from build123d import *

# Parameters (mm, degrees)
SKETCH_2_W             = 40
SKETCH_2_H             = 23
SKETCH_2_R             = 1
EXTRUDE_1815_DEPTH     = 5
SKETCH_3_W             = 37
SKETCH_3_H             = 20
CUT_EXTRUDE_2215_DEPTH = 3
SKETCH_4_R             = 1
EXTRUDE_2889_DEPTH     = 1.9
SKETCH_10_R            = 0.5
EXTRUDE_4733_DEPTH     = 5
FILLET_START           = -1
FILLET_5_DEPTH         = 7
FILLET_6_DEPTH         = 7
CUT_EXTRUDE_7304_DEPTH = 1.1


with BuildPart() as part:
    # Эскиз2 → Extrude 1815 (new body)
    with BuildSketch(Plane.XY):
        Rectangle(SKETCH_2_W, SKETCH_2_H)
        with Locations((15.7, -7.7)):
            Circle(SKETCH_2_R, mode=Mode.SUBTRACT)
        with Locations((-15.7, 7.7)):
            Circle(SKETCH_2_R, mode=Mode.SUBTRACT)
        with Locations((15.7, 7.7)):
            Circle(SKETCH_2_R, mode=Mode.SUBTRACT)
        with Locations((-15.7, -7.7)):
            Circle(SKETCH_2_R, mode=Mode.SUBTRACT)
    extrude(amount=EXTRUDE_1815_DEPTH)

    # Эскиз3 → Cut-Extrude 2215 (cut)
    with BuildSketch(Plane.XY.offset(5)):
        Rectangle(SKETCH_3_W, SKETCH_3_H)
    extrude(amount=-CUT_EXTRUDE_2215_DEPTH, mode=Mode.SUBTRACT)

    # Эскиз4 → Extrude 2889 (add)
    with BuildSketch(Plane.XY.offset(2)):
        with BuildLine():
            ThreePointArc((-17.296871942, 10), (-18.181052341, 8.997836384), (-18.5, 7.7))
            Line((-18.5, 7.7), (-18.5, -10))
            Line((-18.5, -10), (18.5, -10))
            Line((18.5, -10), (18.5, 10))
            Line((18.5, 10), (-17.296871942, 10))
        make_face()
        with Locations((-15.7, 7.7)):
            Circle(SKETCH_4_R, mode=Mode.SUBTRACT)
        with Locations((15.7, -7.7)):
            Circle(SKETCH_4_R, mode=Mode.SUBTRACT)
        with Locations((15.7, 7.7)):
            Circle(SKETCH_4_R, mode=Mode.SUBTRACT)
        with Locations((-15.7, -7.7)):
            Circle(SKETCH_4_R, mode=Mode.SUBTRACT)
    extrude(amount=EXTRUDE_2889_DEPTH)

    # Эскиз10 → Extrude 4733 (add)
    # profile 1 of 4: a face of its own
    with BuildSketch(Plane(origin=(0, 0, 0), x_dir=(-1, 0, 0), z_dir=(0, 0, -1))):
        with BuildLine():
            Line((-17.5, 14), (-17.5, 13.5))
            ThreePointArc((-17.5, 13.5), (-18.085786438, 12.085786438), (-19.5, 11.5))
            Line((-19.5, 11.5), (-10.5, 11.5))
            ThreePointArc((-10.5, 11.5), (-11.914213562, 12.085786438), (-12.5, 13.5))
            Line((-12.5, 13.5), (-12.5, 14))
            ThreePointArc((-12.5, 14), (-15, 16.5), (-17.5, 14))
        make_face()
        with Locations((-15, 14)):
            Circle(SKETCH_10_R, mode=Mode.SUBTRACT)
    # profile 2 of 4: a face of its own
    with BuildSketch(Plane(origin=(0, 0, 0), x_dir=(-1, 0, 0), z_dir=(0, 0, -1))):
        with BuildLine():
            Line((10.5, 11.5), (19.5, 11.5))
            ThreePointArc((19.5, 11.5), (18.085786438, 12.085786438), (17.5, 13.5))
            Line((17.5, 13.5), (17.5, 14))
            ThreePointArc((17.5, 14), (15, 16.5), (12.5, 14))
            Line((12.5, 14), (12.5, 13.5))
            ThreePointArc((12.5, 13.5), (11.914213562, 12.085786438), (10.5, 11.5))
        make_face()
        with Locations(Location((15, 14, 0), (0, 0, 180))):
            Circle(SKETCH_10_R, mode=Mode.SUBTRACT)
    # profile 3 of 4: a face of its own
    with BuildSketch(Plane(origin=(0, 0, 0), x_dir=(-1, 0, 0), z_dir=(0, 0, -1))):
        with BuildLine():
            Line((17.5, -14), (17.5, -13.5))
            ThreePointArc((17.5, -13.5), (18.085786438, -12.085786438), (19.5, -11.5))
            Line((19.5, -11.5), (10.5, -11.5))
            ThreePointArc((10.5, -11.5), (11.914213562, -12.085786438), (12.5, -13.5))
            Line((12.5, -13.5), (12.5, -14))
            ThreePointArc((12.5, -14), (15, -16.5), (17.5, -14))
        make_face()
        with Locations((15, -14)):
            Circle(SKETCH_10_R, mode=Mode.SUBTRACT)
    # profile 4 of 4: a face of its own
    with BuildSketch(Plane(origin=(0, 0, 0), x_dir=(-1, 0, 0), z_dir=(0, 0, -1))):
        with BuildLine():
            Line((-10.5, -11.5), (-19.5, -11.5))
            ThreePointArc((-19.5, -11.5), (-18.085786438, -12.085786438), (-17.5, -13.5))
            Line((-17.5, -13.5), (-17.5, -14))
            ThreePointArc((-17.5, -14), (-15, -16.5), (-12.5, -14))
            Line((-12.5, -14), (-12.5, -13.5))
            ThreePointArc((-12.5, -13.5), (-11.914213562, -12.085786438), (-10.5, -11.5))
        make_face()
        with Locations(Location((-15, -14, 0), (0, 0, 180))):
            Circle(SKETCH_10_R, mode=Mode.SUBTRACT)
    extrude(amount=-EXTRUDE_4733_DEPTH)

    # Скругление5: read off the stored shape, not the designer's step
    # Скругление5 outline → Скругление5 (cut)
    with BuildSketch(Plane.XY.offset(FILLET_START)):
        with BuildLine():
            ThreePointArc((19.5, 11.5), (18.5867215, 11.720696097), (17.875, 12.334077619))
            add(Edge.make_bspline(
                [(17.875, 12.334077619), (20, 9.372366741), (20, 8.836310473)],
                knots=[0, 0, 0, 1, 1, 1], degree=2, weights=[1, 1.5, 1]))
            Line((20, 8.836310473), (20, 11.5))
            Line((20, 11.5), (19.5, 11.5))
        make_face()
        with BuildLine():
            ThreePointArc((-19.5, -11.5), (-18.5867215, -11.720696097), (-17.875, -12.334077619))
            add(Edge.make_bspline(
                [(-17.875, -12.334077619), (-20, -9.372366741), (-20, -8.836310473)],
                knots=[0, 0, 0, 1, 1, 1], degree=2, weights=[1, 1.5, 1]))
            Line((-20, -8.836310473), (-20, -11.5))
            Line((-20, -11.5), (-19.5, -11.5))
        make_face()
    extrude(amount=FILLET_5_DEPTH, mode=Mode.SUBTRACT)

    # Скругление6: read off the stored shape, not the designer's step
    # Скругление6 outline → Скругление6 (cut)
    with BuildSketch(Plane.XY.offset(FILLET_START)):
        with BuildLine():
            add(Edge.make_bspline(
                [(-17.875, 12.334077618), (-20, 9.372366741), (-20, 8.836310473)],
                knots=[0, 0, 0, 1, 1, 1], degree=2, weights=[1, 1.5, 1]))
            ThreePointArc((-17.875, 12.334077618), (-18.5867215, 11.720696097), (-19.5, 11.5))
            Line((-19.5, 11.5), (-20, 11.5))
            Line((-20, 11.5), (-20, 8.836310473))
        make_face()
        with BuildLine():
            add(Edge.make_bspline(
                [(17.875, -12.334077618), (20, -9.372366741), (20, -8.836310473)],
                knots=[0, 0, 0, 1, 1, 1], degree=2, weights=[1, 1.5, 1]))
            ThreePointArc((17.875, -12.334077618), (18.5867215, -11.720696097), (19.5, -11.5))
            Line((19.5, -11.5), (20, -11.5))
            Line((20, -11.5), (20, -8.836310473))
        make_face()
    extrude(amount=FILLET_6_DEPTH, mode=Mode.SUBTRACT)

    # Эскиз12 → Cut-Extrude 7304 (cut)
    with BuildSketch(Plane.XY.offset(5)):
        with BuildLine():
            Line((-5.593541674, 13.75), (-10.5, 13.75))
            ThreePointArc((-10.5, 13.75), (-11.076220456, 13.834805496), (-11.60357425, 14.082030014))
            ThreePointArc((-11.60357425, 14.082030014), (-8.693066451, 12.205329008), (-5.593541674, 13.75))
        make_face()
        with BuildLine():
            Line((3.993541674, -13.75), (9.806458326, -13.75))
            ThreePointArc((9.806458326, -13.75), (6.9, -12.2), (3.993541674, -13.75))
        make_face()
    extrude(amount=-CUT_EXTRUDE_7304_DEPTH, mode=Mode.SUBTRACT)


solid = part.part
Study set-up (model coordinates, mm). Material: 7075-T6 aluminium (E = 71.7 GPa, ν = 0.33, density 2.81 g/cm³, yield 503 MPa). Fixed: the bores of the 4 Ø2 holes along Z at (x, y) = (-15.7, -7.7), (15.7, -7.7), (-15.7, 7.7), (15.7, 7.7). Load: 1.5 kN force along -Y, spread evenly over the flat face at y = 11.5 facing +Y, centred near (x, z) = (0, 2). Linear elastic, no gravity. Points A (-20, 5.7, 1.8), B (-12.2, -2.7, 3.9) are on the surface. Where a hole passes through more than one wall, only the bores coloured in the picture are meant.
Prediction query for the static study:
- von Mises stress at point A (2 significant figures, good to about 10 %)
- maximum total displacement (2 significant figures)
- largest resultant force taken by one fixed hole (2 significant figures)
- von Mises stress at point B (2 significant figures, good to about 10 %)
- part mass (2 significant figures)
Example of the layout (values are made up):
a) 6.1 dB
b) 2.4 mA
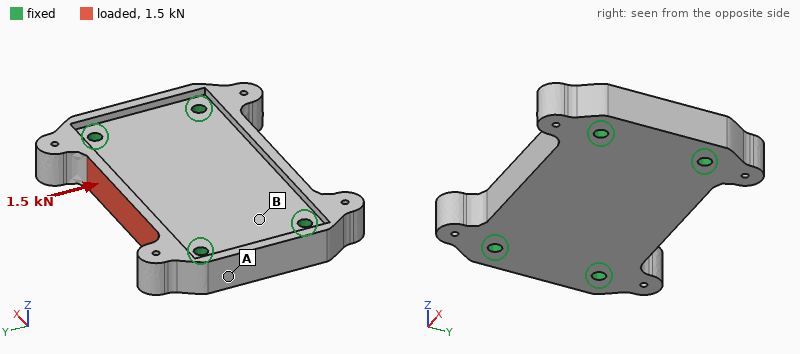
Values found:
a) 6.2 MPa
b) 11 µm
c) 450 N
d) 19 MPa
e) 12 g
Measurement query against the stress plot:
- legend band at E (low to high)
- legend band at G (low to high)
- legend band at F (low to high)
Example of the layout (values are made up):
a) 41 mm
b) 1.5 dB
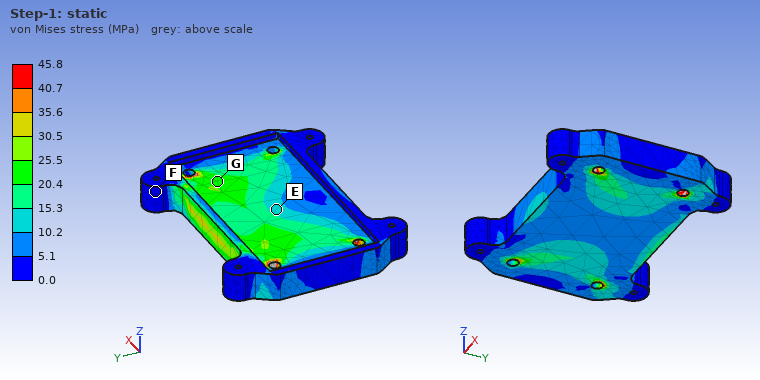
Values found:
a) 10.2 to 15.3 MPa
b) 20.4 to 25.5 MPa
c) 0.0 to 5.1 MPa
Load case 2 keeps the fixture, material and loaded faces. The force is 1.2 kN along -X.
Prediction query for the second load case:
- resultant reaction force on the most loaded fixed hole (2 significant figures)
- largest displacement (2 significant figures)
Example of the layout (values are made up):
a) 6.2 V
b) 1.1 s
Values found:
a) 510 N
b) 4.0 µm
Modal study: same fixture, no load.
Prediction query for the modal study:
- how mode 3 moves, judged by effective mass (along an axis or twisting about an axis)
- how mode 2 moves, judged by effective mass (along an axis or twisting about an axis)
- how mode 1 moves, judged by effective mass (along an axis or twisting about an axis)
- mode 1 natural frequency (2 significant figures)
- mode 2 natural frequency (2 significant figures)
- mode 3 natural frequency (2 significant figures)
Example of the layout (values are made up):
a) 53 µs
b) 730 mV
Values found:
a) along Y
b) twisting about X
c) along Z
d) 18 kHz
e) 24 kHz
f) 39 kHz
